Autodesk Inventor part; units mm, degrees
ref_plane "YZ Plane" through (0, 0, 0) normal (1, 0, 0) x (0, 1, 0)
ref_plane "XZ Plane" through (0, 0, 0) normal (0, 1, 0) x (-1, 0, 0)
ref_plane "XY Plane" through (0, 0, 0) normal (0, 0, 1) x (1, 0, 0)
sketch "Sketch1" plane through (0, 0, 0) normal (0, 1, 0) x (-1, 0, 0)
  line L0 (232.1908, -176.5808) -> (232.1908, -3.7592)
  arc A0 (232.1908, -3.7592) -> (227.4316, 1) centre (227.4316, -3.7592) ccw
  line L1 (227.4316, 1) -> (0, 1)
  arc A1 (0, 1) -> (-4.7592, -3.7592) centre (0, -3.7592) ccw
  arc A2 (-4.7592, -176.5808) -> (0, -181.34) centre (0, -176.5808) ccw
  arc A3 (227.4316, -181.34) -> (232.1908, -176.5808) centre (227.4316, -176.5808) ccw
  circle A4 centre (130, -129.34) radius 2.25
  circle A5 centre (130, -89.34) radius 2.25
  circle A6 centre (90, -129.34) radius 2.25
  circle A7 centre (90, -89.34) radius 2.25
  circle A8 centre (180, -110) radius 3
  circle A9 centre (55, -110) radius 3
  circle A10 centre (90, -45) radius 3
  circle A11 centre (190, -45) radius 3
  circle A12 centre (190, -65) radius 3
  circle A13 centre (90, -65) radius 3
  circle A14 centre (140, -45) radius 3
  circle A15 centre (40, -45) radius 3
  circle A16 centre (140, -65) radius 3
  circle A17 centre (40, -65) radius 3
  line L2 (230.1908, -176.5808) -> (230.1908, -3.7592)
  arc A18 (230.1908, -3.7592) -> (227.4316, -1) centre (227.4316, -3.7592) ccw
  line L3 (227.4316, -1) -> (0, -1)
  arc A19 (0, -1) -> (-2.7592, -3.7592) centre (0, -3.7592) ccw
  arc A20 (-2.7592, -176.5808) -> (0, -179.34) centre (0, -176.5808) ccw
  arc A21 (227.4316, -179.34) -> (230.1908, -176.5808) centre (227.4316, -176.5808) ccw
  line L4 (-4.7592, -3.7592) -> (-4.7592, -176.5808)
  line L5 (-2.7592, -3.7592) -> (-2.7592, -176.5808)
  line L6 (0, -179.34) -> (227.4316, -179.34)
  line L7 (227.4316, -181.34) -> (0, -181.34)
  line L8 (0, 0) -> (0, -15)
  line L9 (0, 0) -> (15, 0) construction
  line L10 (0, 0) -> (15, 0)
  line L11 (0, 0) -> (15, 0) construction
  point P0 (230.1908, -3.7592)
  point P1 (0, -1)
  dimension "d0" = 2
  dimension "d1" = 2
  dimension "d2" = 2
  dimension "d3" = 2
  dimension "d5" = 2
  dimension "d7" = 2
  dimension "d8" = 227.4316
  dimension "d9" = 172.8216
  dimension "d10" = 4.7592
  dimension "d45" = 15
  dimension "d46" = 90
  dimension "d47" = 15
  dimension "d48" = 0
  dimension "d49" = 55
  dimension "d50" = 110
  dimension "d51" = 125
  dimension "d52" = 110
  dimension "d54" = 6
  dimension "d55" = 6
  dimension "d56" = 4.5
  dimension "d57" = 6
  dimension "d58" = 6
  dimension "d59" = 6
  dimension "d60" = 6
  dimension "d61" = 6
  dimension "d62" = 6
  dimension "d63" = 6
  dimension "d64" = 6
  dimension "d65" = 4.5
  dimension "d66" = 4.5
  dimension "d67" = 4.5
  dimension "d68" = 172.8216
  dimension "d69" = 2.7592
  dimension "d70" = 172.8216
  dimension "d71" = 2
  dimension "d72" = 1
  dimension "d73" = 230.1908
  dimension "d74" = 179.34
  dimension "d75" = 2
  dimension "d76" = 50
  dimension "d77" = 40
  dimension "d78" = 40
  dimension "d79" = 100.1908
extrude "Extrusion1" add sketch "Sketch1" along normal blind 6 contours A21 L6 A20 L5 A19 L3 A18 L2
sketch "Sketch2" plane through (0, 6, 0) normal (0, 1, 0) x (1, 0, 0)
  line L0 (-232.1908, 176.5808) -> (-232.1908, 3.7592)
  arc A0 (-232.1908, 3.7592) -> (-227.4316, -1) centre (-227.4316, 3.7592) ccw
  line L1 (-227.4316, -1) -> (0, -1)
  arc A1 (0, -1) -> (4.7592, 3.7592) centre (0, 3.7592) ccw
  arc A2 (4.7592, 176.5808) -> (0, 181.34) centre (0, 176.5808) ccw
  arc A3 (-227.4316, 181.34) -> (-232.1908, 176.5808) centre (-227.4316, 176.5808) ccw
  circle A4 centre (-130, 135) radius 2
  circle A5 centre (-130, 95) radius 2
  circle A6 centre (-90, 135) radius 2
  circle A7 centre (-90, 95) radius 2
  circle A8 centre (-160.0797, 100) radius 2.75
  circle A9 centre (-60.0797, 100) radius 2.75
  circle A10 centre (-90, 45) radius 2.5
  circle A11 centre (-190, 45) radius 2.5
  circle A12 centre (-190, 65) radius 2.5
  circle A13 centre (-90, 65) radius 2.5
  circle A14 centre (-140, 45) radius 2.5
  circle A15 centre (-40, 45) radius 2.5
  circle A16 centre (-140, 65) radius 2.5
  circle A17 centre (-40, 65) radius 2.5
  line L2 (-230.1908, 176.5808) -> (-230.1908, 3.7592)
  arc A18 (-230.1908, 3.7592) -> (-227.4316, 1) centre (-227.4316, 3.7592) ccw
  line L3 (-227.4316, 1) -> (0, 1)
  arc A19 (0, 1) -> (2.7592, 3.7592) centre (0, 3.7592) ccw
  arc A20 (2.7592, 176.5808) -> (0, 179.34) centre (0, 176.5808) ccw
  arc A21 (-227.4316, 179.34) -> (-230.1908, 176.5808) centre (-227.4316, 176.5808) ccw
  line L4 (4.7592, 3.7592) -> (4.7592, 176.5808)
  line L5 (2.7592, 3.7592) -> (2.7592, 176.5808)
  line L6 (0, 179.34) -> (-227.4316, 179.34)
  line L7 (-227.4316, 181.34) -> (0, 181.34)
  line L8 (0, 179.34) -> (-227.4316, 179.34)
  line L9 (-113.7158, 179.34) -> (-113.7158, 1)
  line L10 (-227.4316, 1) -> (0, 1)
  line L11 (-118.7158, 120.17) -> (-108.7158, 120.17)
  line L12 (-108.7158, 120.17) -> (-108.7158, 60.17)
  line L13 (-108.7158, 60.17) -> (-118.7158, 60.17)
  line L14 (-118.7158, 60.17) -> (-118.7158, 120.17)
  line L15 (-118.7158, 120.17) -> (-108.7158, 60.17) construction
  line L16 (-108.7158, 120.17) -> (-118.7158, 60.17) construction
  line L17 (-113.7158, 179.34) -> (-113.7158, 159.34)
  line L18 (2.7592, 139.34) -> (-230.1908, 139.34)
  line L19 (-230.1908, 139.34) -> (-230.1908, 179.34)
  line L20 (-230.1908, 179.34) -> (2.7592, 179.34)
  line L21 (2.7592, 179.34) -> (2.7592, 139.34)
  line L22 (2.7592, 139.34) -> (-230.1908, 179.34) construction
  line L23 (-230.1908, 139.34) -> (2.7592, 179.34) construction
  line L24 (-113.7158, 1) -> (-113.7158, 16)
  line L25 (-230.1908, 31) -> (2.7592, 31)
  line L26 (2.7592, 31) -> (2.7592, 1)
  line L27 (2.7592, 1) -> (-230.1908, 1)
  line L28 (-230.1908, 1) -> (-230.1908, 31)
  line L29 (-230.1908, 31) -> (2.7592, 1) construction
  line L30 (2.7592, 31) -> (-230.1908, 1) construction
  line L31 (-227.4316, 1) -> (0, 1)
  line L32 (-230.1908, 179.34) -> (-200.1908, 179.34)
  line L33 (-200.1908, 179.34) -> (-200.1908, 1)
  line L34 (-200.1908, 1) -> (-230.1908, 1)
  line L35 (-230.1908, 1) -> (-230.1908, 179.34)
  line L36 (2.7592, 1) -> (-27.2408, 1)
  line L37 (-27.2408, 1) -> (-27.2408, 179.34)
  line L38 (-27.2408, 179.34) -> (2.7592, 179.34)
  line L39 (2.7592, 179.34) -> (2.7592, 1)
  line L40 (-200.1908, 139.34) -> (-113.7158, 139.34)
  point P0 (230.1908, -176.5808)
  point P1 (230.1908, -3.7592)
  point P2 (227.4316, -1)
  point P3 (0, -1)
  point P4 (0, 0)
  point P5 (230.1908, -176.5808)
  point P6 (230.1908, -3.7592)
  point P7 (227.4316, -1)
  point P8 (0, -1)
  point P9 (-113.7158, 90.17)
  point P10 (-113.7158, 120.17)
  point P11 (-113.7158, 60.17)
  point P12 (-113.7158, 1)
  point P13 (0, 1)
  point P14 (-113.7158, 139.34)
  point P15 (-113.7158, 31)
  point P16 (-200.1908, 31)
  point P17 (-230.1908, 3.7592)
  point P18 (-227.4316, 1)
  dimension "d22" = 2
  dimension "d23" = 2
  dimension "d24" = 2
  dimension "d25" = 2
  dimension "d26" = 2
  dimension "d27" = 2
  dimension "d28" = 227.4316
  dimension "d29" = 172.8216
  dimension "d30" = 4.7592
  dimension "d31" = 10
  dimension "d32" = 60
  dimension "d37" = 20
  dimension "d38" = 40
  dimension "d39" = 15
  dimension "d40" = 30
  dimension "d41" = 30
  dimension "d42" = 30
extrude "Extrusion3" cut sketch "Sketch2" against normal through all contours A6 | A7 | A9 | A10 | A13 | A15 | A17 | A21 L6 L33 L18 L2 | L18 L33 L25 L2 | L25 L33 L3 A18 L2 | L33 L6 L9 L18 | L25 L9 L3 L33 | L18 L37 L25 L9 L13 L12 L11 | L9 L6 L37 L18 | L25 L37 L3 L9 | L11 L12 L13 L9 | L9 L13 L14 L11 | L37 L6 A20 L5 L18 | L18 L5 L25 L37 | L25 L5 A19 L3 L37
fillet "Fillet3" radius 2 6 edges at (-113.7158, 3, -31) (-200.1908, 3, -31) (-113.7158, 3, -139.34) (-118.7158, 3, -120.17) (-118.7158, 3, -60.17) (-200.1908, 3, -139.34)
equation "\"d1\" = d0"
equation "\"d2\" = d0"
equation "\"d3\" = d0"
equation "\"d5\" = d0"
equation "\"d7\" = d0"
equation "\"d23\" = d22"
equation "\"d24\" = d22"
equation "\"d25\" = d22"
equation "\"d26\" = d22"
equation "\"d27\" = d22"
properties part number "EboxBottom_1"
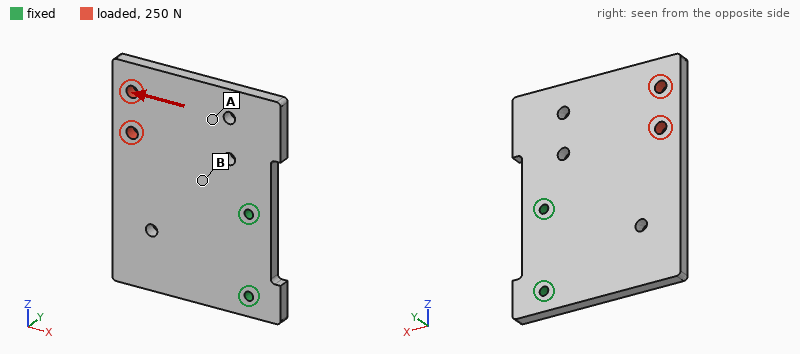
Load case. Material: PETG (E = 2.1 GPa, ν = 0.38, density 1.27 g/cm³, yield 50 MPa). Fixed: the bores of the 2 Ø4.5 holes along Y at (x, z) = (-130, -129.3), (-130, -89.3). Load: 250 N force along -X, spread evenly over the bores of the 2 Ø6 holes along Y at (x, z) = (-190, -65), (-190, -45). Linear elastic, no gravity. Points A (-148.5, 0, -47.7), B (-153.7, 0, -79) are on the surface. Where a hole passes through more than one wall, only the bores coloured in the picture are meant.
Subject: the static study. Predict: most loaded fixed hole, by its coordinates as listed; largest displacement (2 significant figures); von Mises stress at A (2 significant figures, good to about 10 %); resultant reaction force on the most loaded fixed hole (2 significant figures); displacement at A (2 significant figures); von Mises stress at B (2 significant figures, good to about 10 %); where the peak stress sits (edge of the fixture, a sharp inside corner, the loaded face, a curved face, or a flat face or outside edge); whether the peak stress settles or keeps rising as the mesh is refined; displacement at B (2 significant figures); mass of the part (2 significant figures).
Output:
(-130, -89.3)
0.22 mm
0.65 MPa
450 N
0.14 mm
1.6 MPa
edge of the fixture
keeps rising
0.067 mm
68 g
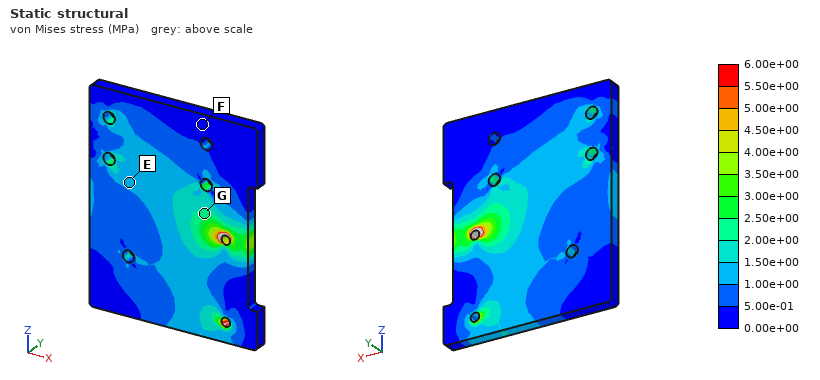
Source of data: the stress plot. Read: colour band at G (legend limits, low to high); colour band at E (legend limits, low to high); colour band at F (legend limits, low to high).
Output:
2.00e+00 to 2.50e+00 MPa
1.00e+00 to 1.50e+00 MPa
0.00e+00 to 5.00e-01 MPa
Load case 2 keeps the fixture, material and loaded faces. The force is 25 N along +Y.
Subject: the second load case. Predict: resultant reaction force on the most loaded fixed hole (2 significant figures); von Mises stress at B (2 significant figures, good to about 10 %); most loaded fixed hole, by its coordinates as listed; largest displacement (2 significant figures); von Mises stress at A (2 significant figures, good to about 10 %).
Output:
39 N
2.0 MPa
(-130, -89.3)
1.6 mm
1.3 MPa
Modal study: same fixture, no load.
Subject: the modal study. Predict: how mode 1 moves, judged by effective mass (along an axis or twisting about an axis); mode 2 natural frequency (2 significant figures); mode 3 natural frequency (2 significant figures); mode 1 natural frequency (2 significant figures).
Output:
along Y
290 Hz
530 Hz
190 Hz
